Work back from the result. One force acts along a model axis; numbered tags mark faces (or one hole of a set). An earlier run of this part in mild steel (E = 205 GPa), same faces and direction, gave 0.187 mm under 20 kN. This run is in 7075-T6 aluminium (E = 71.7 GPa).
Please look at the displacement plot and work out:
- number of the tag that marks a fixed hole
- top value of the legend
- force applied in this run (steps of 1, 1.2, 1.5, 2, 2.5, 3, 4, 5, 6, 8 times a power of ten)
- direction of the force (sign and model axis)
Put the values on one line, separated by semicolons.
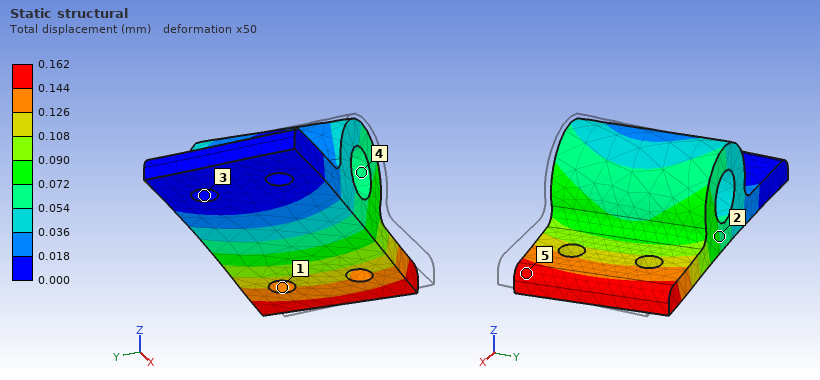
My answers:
3; 0.162 mm; 6 kN; +Y
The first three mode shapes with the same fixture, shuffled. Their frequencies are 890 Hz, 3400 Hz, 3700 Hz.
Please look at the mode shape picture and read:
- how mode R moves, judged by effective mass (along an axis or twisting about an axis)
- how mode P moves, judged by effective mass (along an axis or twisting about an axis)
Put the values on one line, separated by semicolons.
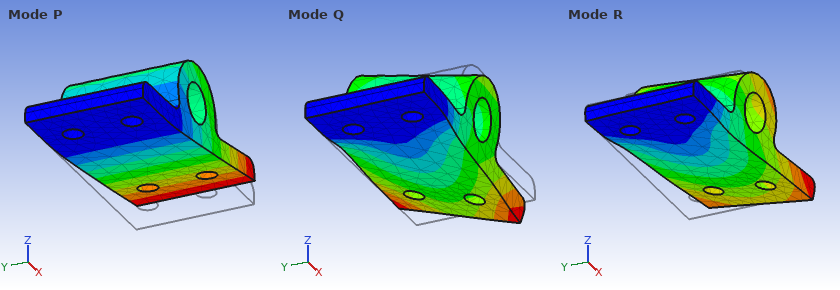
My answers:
along Y; along Z
